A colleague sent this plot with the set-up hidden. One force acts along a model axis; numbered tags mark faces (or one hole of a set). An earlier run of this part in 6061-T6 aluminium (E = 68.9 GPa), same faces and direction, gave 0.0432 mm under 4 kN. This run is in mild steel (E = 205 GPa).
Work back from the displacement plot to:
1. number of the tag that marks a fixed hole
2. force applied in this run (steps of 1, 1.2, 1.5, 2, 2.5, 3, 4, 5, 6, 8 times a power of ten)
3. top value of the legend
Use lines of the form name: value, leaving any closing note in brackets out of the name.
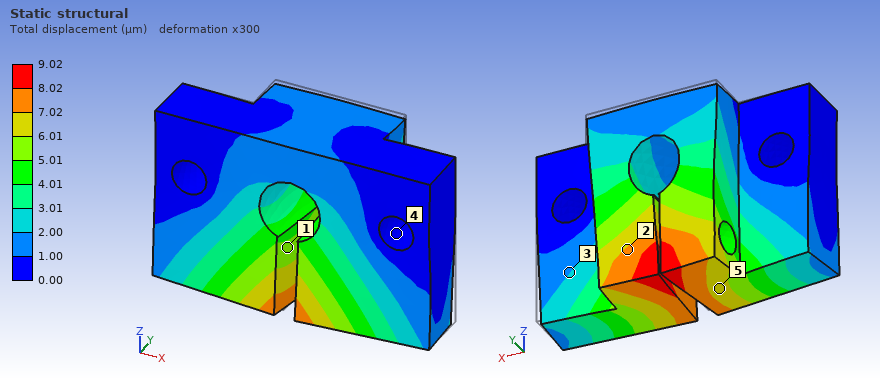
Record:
number of the tag that marks a fixed hole: 4
force applied in this run: 2.5 kN
top value of the legend: 9.02 µm
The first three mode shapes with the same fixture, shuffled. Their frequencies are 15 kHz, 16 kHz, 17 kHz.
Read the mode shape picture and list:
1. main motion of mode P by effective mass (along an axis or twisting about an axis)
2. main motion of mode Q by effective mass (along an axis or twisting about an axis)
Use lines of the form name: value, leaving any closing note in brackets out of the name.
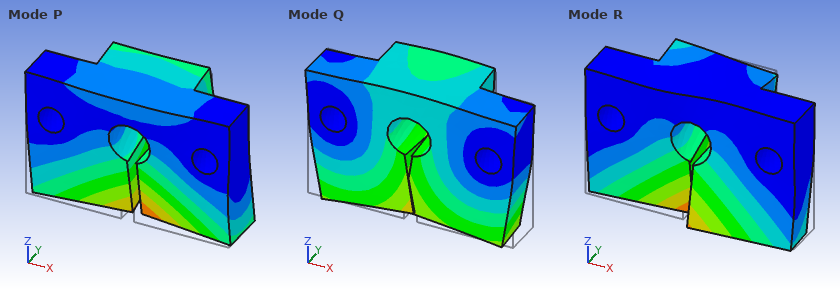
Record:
main motion of mode P by effective mass: along Y
main motion of mode Q by effective mass: along Z
